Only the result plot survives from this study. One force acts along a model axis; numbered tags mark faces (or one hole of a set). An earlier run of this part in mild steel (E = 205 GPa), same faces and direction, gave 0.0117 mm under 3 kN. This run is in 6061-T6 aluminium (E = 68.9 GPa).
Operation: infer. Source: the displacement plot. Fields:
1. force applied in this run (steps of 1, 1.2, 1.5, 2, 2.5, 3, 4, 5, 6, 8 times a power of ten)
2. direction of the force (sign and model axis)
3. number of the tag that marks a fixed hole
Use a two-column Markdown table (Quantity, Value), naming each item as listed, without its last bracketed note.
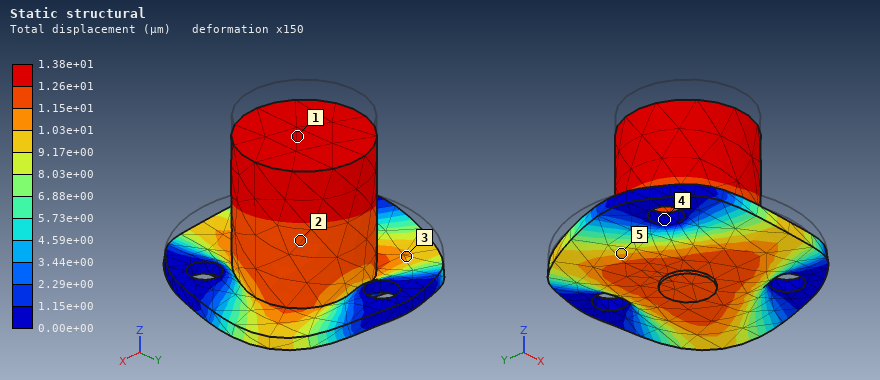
| Quantity | Value |
|---|---|
| force applied in this run | 1.2 kN |
| direction of the force | -Z |
| number of the tag that marks a fixed hole | 4 |
